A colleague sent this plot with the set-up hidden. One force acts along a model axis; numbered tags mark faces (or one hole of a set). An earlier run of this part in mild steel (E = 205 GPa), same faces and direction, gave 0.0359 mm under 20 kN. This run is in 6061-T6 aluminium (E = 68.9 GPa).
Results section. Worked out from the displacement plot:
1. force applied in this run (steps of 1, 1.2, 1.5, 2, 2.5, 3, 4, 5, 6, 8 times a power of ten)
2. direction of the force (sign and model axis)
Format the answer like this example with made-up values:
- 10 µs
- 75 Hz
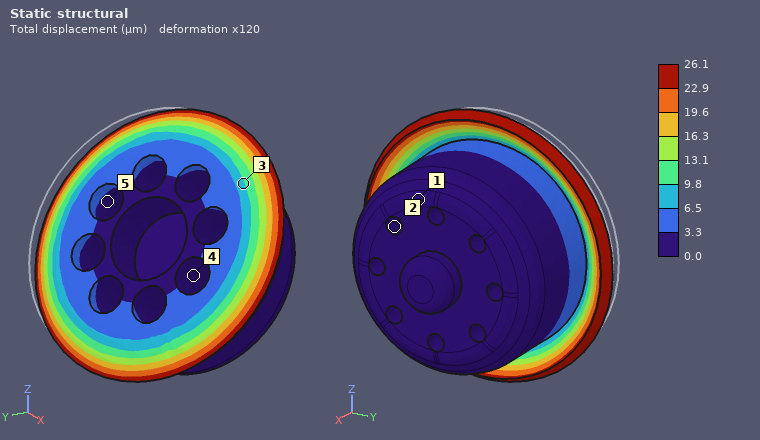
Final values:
- 5 kN
- +X
